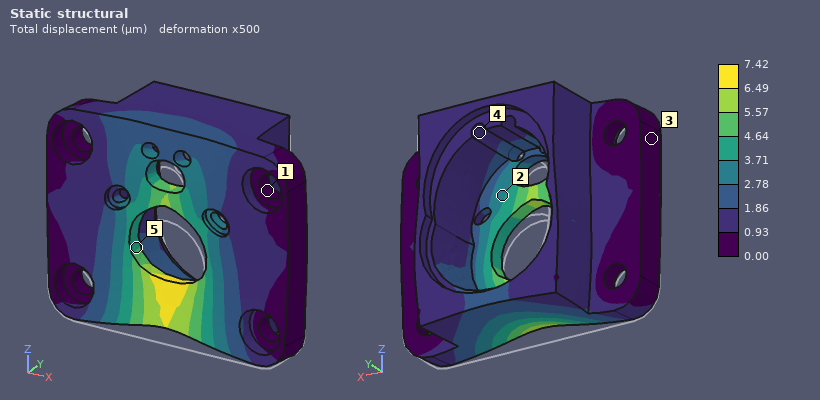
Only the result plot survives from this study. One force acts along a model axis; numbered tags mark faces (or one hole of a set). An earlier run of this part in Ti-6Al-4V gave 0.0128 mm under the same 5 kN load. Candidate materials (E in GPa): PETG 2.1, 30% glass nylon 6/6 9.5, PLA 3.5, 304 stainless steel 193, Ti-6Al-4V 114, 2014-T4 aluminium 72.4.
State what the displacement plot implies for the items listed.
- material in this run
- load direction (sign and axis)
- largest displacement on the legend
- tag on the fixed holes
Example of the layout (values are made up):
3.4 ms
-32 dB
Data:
304 stainless steel
+Z
7.42 µm
1
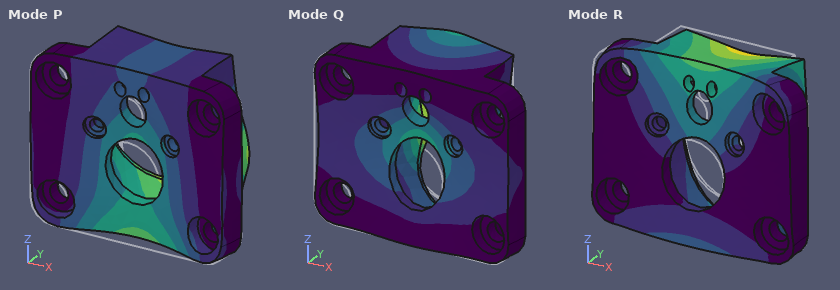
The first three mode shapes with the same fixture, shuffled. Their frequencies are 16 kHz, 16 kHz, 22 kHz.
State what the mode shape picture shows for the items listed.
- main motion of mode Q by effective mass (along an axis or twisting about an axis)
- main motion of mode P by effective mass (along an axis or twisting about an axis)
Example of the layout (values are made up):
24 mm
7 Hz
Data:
along Y
along Y
